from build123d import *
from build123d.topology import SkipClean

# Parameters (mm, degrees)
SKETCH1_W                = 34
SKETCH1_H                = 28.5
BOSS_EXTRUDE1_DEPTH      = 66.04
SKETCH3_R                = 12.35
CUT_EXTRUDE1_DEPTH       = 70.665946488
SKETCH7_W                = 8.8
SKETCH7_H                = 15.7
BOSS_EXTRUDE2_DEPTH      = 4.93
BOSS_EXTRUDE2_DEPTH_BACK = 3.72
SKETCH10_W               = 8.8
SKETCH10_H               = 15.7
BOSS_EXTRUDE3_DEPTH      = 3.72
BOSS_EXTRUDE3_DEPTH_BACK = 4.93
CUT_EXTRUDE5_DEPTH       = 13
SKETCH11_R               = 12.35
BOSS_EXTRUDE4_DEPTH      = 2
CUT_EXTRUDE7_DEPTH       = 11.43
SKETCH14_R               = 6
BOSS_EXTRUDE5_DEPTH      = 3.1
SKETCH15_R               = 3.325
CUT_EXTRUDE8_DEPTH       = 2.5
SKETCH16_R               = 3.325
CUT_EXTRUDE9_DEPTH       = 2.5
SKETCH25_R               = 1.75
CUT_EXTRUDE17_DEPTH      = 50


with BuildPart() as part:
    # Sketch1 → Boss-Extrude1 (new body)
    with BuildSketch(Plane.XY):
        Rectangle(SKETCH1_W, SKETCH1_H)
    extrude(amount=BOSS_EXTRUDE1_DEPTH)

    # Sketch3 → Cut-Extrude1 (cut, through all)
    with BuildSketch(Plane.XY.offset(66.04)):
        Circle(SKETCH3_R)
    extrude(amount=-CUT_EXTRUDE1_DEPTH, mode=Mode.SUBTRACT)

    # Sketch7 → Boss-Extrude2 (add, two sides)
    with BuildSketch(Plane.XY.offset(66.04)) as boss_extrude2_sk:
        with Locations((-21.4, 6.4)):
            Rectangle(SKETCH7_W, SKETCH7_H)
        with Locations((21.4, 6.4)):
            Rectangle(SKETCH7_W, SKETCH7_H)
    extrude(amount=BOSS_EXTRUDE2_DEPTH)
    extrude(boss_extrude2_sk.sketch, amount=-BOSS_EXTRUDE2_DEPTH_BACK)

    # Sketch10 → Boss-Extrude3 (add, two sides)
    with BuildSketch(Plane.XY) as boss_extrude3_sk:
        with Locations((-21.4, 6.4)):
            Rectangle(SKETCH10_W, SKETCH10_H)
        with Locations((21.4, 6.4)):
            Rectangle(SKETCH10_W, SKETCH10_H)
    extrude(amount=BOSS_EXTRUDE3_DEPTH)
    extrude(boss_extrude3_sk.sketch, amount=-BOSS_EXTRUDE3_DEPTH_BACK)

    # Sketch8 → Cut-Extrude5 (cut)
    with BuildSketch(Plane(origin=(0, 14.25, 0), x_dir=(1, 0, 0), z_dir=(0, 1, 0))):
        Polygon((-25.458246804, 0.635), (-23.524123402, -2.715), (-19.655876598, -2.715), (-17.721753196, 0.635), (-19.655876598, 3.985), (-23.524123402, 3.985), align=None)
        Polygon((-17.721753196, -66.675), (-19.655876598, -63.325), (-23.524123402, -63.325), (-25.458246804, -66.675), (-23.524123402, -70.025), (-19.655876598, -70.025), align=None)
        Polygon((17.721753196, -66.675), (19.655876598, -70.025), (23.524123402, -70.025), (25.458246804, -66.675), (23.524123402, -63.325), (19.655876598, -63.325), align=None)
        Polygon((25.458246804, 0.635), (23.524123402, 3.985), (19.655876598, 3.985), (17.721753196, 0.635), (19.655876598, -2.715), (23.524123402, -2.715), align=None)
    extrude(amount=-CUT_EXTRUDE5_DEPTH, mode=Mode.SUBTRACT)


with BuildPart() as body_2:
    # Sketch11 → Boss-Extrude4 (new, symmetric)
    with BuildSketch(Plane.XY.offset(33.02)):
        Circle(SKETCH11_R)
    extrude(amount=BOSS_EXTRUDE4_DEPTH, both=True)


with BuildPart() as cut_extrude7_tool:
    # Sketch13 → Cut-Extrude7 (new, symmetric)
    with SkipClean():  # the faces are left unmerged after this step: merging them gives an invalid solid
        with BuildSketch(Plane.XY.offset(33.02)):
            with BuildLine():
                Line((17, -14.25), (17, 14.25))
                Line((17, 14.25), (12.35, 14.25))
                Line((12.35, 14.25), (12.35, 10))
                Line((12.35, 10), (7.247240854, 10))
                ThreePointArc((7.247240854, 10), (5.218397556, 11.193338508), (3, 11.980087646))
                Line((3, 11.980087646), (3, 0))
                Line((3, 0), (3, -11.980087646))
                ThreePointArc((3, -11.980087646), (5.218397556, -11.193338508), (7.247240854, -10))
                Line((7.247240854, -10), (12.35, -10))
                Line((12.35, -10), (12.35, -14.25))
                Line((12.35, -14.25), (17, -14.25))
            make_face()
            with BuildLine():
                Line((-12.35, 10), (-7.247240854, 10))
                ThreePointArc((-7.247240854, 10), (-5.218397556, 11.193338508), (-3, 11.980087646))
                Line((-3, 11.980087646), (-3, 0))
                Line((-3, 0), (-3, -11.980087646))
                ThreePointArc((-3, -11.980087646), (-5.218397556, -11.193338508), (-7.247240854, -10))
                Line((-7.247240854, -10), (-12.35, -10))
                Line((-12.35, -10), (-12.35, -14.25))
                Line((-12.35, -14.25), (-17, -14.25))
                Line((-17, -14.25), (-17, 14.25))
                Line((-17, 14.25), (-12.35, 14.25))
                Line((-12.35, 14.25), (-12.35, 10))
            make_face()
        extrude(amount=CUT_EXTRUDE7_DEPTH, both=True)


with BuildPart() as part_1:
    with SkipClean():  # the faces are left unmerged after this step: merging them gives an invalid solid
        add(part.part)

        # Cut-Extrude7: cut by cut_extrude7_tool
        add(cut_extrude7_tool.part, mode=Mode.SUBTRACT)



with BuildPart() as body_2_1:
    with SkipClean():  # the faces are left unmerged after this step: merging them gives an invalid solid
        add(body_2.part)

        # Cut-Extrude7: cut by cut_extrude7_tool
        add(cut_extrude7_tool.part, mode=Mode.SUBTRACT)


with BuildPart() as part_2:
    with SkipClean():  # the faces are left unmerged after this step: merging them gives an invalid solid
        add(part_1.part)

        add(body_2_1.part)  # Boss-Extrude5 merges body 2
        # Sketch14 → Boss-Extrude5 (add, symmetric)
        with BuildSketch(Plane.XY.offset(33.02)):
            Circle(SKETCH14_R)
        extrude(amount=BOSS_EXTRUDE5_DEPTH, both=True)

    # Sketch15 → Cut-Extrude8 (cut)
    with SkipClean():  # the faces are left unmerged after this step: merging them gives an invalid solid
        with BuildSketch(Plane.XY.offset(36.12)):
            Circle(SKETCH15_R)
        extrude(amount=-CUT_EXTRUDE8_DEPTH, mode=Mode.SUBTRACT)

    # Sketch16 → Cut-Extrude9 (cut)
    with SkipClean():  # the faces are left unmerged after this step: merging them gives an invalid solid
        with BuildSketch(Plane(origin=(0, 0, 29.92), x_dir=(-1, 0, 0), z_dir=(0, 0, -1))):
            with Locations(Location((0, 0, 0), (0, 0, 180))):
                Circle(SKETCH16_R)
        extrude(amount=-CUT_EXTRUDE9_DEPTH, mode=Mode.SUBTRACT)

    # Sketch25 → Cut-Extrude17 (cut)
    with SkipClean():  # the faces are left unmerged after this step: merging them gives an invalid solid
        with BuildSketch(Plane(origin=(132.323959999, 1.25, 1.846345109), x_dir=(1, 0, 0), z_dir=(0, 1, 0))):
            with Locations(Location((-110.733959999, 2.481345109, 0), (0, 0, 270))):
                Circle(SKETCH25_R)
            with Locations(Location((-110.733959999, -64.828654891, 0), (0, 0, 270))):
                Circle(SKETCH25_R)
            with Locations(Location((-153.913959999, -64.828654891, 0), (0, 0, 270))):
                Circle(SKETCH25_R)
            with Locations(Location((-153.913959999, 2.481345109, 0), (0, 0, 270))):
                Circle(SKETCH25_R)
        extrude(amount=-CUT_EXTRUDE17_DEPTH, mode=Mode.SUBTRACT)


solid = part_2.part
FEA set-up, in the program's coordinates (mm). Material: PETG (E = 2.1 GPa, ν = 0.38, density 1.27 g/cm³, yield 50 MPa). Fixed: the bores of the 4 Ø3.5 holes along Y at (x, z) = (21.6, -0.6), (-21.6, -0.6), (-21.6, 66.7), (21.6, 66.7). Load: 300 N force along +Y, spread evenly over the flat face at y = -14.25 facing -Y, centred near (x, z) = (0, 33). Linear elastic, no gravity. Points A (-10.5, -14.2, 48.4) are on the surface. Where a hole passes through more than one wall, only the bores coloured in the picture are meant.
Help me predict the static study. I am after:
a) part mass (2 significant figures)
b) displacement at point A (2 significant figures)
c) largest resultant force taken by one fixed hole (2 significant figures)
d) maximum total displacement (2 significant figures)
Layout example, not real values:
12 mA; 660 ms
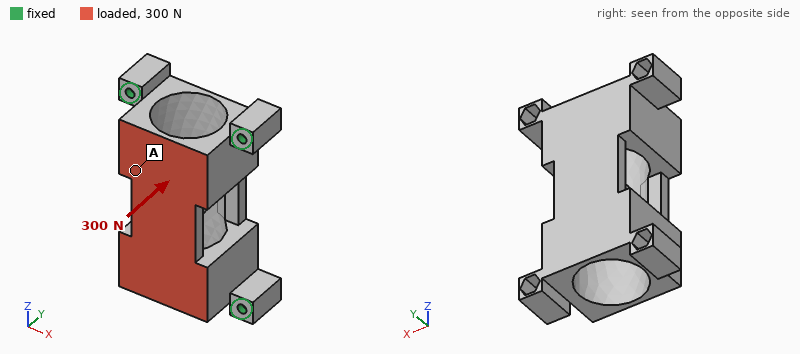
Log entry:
36 g; 51 µm; 75 N; 79 µm
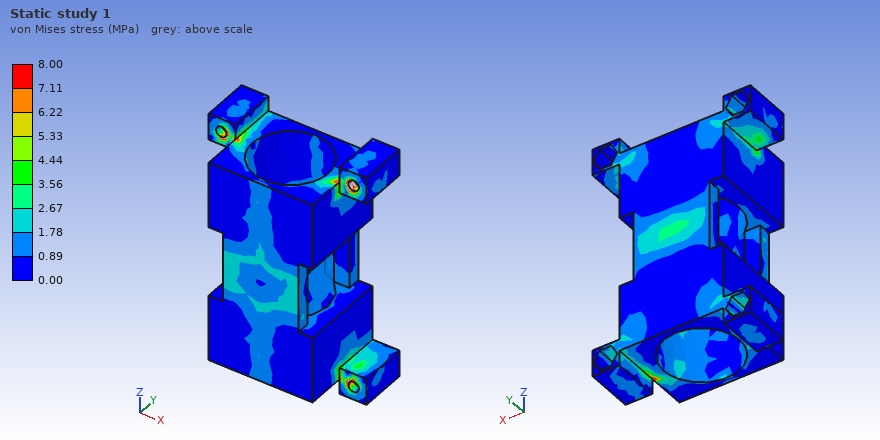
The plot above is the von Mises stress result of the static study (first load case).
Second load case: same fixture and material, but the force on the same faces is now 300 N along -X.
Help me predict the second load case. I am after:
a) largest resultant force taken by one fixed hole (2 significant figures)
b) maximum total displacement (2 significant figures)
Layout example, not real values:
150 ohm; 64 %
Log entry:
100 N; 0.13 mm
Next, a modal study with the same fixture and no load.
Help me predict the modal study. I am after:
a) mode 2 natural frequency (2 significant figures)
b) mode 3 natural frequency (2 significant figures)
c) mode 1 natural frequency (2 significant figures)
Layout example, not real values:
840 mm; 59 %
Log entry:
2200 Hz; 2200 Hz; 2000 Hz
